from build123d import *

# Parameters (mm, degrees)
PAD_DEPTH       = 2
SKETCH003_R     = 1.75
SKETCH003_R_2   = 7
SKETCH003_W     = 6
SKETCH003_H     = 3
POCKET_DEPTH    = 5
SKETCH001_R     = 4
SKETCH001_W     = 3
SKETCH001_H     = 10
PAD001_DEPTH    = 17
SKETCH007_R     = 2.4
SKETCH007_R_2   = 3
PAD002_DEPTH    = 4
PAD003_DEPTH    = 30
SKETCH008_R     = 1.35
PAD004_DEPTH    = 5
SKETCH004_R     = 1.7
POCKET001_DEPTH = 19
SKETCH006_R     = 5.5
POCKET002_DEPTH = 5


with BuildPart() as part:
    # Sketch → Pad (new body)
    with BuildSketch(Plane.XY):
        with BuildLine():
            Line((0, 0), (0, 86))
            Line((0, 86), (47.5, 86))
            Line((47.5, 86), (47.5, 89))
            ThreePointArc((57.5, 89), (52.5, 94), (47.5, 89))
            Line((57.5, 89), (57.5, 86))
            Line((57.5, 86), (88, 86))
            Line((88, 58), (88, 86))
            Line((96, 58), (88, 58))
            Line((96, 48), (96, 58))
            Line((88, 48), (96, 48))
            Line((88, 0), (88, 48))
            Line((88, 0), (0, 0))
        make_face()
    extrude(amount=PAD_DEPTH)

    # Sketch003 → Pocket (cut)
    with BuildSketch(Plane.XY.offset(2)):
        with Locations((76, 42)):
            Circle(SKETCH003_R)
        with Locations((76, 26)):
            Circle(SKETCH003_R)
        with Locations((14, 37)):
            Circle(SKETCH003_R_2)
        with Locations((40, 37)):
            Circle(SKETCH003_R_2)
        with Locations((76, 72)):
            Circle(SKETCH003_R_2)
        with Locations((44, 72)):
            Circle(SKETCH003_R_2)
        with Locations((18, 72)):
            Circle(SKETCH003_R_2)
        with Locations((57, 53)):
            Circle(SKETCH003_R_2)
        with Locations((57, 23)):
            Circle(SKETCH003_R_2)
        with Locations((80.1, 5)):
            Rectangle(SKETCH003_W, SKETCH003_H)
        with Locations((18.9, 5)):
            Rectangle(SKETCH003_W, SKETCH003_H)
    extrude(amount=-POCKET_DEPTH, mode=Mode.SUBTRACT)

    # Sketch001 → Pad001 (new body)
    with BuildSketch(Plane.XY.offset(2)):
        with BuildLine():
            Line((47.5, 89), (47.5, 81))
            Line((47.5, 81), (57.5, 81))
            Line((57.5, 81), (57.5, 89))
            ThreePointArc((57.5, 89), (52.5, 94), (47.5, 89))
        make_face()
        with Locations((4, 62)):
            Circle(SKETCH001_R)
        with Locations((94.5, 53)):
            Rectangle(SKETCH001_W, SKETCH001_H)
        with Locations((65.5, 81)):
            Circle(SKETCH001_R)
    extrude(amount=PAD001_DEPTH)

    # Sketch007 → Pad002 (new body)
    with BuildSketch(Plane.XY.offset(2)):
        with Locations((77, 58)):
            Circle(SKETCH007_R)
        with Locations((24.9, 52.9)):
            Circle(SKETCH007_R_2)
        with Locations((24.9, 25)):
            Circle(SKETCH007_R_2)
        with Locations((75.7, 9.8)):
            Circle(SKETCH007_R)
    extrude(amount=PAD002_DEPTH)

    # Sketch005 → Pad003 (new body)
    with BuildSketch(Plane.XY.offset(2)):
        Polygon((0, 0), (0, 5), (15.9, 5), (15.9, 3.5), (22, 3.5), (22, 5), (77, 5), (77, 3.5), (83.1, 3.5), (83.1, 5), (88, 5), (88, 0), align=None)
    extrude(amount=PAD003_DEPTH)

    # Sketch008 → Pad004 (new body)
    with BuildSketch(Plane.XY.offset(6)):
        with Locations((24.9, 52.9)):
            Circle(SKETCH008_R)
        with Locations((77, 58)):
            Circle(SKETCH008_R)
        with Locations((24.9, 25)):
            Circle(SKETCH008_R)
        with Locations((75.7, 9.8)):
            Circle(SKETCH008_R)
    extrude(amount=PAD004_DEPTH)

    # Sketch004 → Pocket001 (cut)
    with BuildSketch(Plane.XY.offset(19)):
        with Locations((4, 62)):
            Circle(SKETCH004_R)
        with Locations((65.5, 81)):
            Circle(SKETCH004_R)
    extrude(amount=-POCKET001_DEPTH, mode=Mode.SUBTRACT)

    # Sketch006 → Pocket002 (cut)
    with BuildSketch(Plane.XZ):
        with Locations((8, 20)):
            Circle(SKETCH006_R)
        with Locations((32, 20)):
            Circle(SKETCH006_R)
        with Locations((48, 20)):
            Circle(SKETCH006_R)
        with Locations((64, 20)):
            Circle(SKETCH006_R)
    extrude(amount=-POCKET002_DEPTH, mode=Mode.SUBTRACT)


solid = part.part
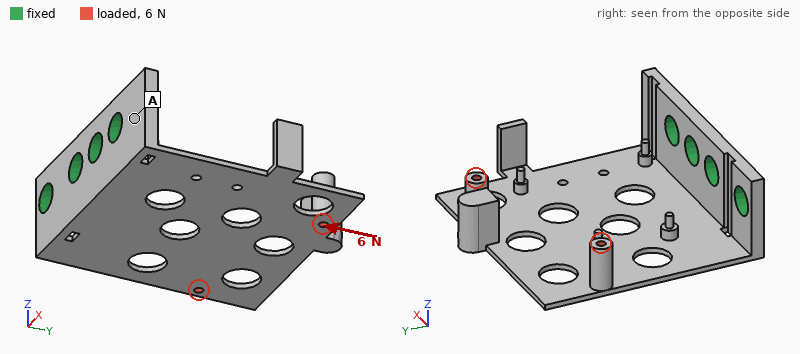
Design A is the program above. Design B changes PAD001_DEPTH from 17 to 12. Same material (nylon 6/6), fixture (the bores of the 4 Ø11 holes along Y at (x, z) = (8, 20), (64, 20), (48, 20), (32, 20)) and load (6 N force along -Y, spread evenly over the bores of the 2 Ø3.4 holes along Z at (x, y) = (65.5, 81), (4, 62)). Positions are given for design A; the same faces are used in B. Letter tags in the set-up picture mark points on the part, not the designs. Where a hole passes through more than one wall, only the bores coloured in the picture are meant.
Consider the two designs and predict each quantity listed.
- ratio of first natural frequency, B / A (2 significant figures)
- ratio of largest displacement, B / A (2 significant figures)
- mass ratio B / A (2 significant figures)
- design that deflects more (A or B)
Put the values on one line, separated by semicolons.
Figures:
1.1; 0.68; 0.96; A
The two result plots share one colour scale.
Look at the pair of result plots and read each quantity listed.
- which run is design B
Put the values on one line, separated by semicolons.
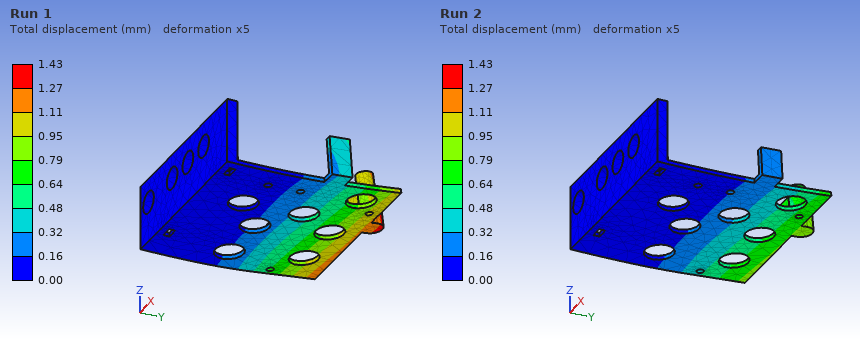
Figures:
Run 2
